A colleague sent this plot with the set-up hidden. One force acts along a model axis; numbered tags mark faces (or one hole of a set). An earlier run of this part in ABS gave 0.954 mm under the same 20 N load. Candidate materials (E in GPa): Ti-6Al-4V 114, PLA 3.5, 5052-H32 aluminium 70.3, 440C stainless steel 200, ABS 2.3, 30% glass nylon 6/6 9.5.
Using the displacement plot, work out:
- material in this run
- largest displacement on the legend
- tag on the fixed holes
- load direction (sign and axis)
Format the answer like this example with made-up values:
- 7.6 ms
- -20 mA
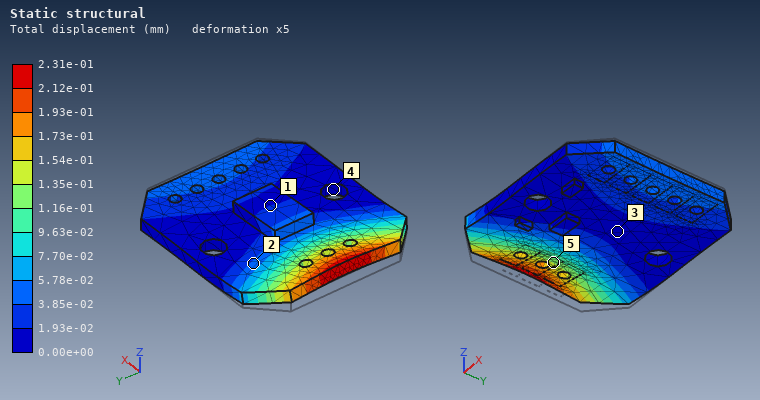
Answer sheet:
- 30% glass nylon 6/6
- 2.31e-01 mm
- 4
- +Z
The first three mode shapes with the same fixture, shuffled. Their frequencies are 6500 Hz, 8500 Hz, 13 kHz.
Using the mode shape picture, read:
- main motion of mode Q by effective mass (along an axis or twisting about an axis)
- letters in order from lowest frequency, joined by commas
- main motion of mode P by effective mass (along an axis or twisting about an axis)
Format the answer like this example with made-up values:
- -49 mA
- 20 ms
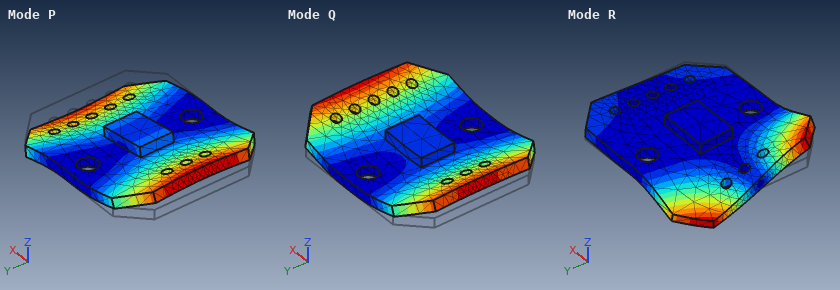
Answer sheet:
- along Z
- P, Q, R
- twisting about Y
